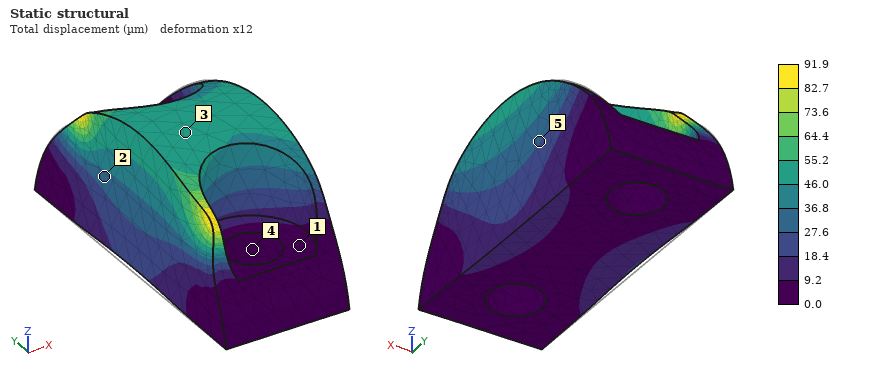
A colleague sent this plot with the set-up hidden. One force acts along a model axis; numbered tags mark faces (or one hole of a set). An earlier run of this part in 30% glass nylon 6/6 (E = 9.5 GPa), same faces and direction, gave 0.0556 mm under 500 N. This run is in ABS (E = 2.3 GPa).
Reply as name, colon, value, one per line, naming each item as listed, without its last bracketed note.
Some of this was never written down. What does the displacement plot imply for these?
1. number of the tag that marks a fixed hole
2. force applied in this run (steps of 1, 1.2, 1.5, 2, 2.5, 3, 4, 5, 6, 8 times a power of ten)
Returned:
number of the tag that marks a fixed hole: 4
force applied in this run: 200 N
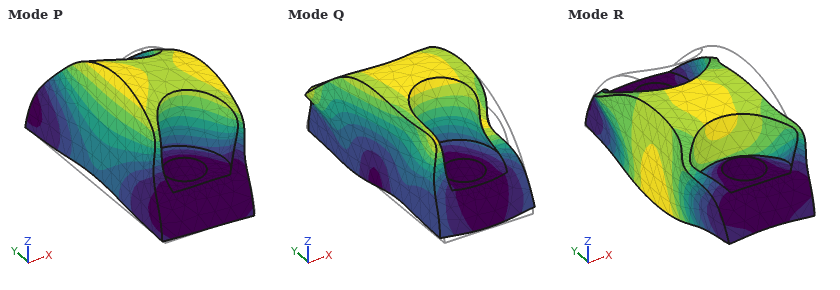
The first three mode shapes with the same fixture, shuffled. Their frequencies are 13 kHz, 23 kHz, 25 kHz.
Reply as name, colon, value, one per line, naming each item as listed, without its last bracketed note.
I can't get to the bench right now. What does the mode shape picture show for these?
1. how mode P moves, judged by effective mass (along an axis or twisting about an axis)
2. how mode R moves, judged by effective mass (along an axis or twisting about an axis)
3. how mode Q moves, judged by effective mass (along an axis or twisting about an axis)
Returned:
how mode P moves, judged by effective mass: along X
how mode R moves, judged by effective mass: along Z
how mode Q moves, judged by effective mass: along Y
